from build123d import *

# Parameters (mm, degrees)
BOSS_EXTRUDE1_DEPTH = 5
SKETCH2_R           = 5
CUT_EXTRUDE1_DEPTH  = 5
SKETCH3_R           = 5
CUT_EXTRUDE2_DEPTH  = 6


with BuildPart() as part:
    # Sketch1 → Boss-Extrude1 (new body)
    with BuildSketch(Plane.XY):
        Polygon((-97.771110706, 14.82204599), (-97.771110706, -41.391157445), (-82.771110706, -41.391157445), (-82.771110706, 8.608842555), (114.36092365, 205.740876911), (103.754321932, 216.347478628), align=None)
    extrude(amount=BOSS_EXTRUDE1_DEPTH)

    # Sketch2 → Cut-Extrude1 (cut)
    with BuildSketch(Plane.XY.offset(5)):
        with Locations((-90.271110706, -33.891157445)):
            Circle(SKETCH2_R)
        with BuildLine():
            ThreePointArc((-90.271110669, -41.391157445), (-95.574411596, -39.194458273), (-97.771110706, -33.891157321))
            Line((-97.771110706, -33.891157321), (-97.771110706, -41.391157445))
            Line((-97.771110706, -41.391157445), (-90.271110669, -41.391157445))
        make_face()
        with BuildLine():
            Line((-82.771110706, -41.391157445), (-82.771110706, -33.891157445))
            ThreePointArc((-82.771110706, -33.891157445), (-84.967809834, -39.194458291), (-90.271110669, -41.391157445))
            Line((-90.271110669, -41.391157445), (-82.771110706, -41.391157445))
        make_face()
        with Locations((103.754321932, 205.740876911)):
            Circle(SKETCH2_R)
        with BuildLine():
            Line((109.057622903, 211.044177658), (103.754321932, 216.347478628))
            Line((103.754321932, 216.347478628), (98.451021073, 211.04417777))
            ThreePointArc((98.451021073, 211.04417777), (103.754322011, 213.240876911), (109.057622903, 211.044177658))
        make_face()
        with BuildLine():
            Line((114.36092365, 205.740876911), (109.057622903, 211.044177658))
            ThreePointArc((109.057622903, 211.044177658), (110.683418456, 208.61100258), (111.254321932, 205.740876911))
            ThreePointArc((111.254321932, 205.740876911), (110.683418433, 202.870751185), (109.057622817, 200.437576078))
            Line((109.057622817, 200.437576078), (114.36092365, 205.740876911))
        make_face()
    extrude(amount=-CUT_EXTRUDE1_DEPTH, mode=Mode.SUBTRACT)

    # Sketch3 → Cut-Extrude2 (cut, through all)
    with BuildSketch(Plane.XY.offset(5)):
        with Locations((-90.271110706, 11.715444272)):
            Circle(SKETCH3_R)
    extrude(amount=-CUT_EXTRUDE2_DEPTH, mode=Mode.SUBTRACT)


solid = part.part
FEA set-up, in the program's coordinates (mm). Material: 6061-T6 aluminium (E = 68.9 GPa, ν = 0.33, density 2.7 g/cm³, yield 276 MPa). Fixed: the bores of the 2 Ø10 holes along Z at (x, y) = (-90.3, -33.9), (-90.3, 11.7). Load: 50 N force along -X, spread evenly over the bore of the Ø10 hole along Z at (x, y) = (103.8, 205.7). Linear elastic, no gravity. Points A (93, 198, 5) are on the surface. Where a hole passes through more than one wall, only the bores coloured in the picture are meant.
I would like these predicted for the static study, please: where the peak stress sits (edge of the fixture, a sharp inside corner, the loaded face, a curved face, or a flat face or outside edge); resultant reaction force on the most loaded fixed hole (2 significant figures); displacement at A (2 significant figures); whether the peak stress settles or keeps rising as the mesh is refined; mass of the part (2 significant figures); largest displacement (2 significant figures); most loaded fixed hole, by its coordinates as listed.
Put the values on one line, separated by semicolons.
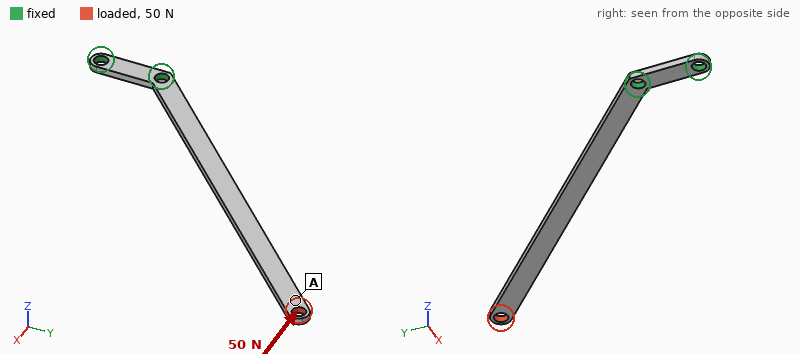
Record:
edge of the fixture; 72 N; 2.3 mm; keeps rising; 64 g; 2.6 mm; (-90.3, 11.7)
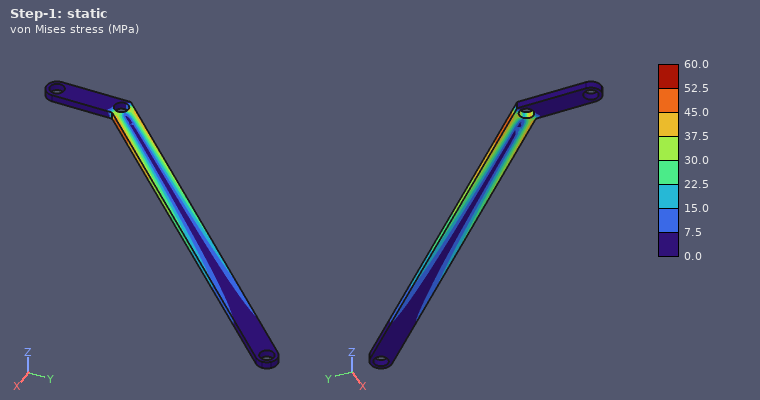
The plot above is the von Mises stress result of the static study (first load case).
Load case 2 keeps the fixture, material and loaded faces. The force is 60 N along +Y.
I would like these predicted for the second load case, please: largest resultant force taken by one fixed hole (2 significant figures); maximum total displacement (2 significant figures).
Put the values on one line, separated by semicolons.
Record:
37 N; 3.1 mm
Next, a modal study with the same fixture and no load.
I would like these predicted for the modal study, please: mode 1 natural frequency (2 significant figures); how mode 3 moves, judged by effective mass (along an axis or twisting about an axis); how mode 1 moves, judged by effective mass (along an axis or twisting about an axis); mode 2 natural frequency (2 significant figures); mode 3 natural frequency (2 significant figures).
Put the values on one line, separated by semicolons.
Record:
56 Hz; along Z; along Z; 160 Hz; 350 Hz
